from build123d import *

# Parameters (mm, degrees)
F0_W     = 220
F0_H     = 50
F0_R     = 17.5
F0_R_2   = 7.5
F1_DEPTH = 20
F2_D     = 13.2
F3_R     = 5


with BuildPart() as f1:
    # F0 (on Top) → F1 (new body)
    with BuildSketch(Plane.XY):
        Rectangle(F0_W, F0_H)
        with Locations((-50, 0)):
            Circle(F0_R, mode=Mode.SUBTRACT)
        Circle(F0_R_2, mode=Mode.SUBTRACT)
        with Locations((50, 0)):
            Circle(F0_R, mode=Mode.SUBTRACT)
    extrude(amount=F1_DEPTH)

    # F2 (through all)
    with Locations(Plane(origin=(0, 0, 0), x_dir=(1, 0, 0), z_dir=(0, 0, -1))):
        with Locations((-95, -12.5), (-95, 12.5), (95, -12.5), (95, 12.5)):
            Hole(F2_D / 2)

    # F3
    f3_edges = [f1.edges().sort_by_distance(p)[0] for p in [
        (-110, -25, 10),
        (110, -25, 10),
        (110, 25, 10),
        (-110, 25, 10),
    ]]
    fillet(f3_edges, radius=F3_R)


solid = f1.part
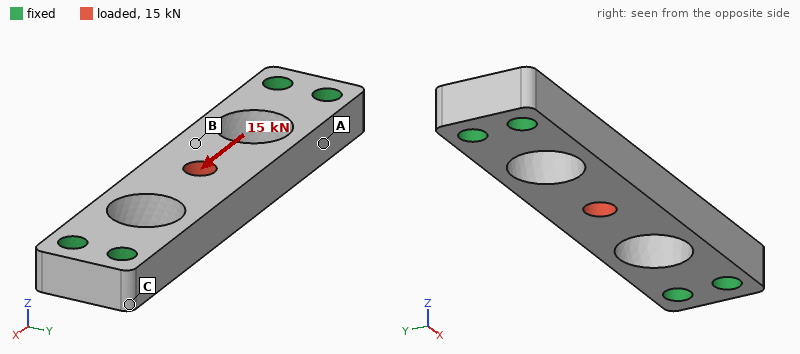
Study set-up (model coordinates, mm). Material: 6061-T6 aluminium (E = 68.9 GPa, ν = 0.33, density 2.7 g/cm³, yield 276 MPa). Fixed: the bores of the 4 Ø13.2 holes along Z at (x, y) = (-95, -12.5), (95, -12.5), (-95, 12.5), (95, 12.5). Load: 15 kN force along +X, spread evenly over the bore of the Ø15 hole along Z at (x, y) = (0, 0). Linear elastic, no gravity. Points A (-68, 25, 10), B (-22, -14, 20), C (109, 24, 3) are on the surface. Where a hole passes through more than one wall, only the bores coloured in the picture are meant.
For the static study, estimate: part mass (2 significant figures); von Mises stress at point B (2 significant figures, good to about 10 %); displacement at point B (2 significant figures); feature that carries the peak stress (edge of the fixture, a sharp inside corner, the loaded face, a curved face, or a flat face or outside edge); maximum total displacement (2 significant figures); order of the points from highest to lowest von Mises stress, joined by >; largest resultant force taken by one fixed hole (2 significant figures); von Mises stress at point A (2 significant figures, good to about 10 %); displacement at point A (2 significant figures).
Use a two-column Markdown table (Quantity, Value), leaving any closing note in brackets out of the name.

| Quantity | Value |
|---|---|
| part mass | 450 g |
| von Mises stress at point B | 13 MPa |
| displacement at point B | 20 µm |
| feature that carries the peak stress | a curved face |
| maximum total displacement | 25 µm |
| order of the points from highest to lowest von Mises stress, joined by > | A > B > C |
| largest resultant force taken by one fixed hole | 3.8 kN |
| von Mises stress at point A | 23 MPa |
| displacement at point A | 7.0 µm |
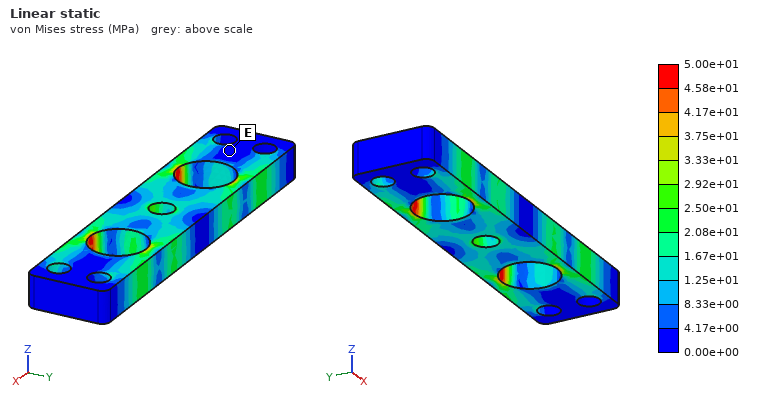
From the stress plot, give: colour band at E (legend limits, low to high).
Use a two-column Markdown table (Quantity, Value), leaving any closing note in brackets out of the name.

| Quantity | Value |
|---|---|
| colour band at E | 0.00e+00 to 4.17e+00 MPa |
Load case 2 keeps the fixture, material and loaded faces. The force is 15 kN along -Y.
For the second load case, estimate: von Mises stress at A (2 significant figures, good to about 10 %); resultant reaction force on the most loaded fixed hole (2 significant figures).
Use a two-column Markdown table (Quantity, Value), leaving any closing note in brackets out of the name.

| Quantity | Value |
|---|---|
| von Mises stress at A | 84 MPa |
| resultant reaction force on the most loaded fixed hole | 10 kN |
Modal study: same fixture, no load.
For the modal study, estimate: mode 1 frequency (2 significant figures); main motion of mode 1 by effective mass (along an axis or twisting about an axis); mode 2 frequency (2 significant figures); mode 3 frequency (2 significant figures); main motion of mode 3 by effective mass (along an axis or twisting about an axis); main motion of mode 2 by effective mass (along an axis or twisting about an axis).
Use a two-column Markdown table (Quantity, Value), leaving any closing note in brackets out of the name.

| Quantity | Value |
|---|---|
| mode 1 frequency | 2800 Hz |
| main motion of mode 1 by effective mass | along Z |
| mode 2 frequency | 3200 Hz |
| mode 3 frequency | 4600 Hz |
| main motion of mode 3 by effective mass | twisting about X |
| main motion of mode 2 by effective mass | along Y |
